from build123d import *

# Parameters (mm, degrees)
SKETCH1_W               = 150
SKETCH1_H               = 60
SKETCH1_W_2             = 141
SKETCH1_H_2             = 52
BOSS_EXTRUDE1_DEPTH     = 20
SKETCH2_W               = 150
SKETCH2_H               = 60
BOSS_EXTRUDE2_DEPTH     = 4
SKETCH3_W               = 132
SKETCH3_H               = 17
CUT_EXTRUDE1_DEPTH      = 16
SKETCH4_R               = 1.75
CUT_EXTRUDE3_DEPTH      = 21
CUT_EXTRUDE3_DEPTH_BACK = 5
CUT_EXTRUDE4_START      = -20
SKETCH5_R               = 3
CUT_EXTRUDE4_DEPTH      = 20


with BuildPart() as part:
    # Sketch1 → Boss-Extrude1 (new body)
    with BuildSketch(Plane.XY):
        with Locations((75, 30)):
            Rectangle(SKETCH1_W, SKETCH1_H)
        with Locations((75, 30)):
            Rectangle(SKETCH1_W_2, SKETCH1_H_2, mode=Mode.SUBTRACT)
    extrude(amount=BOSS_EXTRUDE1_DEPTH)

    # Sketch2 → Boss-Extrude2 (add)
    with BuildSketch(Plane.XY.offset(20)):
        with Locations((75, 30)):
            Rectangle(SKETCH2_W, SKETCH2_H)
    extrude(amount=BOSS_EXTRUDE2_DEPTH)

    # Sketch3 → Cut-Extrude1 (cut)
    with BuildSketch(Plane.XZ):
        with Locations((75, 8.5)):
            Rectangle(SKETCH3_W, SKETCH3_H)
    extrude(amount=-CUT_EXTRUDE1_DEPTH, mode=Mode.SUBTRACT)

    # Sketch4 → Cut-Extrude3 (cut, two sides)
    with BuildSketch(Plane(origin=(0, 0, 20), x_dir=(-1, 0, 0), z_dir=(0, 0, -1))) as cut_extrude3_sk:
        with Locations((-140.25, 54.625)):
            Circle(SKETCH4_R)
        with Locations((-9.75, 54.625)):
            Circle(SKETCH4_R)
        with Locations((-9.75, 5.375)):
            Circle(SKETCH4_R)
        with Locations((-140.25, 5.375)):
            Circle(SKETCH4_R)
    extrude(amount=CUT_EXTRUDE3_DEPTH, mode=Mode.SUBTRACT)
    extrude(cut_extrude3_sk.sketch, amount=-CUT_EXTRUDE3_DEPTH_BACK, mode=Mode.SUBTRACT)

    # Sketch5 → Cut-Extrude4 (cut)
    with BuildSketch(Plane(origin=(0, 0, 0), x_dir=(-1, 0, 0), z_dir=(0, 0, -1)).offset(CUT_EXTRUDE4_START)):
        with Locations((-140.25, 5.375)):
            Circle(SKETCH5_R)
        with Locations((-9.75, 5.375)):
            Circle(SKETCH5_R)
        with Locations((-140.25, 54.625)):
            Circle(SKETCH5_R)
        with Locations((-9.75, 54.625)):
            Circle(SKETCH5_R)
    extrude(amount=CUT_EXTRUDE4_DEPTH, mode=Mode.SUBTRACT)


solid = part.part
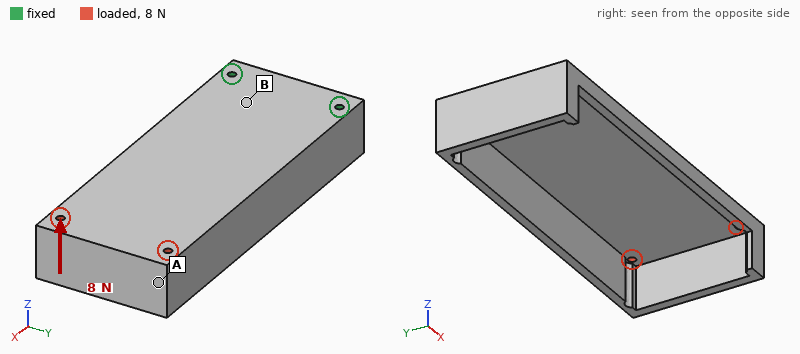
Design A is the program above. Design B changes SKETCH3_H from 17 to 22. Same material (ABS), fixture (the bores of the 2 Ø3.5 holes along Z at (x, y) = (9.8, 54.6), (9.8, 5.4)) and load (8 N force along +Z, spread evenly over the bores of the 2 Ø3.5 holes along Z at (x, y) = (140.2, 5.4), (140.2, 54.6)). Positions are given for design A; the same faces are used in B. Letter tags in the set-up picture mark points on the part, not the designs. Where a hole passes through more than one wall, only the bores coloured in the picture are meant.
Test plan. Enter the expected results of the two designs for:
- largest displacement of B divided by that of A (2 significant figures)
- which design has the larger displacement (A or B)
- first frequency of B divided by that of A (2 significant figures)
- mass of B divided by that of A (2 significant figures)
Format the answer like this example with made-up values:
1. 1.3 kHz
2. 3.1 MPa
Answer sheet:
1. 1.1
2. B
3. 0.96
4. 0.98
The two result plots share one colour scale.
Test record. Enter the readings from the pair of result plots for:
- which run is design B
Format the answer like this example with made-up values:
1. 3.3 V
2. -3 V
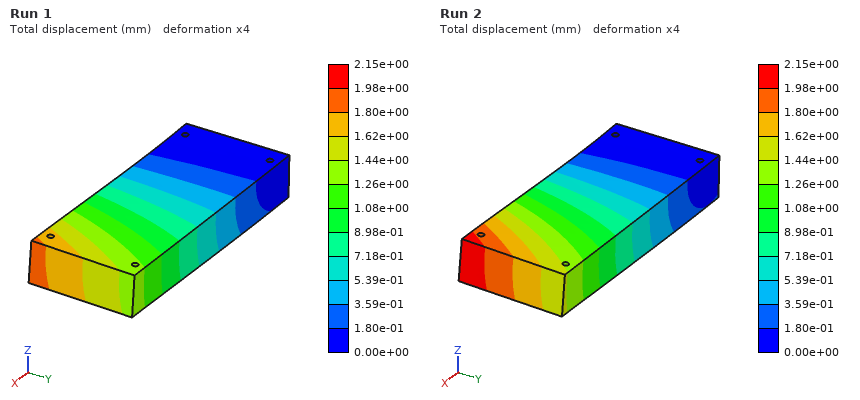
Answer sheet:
1. Run 2
